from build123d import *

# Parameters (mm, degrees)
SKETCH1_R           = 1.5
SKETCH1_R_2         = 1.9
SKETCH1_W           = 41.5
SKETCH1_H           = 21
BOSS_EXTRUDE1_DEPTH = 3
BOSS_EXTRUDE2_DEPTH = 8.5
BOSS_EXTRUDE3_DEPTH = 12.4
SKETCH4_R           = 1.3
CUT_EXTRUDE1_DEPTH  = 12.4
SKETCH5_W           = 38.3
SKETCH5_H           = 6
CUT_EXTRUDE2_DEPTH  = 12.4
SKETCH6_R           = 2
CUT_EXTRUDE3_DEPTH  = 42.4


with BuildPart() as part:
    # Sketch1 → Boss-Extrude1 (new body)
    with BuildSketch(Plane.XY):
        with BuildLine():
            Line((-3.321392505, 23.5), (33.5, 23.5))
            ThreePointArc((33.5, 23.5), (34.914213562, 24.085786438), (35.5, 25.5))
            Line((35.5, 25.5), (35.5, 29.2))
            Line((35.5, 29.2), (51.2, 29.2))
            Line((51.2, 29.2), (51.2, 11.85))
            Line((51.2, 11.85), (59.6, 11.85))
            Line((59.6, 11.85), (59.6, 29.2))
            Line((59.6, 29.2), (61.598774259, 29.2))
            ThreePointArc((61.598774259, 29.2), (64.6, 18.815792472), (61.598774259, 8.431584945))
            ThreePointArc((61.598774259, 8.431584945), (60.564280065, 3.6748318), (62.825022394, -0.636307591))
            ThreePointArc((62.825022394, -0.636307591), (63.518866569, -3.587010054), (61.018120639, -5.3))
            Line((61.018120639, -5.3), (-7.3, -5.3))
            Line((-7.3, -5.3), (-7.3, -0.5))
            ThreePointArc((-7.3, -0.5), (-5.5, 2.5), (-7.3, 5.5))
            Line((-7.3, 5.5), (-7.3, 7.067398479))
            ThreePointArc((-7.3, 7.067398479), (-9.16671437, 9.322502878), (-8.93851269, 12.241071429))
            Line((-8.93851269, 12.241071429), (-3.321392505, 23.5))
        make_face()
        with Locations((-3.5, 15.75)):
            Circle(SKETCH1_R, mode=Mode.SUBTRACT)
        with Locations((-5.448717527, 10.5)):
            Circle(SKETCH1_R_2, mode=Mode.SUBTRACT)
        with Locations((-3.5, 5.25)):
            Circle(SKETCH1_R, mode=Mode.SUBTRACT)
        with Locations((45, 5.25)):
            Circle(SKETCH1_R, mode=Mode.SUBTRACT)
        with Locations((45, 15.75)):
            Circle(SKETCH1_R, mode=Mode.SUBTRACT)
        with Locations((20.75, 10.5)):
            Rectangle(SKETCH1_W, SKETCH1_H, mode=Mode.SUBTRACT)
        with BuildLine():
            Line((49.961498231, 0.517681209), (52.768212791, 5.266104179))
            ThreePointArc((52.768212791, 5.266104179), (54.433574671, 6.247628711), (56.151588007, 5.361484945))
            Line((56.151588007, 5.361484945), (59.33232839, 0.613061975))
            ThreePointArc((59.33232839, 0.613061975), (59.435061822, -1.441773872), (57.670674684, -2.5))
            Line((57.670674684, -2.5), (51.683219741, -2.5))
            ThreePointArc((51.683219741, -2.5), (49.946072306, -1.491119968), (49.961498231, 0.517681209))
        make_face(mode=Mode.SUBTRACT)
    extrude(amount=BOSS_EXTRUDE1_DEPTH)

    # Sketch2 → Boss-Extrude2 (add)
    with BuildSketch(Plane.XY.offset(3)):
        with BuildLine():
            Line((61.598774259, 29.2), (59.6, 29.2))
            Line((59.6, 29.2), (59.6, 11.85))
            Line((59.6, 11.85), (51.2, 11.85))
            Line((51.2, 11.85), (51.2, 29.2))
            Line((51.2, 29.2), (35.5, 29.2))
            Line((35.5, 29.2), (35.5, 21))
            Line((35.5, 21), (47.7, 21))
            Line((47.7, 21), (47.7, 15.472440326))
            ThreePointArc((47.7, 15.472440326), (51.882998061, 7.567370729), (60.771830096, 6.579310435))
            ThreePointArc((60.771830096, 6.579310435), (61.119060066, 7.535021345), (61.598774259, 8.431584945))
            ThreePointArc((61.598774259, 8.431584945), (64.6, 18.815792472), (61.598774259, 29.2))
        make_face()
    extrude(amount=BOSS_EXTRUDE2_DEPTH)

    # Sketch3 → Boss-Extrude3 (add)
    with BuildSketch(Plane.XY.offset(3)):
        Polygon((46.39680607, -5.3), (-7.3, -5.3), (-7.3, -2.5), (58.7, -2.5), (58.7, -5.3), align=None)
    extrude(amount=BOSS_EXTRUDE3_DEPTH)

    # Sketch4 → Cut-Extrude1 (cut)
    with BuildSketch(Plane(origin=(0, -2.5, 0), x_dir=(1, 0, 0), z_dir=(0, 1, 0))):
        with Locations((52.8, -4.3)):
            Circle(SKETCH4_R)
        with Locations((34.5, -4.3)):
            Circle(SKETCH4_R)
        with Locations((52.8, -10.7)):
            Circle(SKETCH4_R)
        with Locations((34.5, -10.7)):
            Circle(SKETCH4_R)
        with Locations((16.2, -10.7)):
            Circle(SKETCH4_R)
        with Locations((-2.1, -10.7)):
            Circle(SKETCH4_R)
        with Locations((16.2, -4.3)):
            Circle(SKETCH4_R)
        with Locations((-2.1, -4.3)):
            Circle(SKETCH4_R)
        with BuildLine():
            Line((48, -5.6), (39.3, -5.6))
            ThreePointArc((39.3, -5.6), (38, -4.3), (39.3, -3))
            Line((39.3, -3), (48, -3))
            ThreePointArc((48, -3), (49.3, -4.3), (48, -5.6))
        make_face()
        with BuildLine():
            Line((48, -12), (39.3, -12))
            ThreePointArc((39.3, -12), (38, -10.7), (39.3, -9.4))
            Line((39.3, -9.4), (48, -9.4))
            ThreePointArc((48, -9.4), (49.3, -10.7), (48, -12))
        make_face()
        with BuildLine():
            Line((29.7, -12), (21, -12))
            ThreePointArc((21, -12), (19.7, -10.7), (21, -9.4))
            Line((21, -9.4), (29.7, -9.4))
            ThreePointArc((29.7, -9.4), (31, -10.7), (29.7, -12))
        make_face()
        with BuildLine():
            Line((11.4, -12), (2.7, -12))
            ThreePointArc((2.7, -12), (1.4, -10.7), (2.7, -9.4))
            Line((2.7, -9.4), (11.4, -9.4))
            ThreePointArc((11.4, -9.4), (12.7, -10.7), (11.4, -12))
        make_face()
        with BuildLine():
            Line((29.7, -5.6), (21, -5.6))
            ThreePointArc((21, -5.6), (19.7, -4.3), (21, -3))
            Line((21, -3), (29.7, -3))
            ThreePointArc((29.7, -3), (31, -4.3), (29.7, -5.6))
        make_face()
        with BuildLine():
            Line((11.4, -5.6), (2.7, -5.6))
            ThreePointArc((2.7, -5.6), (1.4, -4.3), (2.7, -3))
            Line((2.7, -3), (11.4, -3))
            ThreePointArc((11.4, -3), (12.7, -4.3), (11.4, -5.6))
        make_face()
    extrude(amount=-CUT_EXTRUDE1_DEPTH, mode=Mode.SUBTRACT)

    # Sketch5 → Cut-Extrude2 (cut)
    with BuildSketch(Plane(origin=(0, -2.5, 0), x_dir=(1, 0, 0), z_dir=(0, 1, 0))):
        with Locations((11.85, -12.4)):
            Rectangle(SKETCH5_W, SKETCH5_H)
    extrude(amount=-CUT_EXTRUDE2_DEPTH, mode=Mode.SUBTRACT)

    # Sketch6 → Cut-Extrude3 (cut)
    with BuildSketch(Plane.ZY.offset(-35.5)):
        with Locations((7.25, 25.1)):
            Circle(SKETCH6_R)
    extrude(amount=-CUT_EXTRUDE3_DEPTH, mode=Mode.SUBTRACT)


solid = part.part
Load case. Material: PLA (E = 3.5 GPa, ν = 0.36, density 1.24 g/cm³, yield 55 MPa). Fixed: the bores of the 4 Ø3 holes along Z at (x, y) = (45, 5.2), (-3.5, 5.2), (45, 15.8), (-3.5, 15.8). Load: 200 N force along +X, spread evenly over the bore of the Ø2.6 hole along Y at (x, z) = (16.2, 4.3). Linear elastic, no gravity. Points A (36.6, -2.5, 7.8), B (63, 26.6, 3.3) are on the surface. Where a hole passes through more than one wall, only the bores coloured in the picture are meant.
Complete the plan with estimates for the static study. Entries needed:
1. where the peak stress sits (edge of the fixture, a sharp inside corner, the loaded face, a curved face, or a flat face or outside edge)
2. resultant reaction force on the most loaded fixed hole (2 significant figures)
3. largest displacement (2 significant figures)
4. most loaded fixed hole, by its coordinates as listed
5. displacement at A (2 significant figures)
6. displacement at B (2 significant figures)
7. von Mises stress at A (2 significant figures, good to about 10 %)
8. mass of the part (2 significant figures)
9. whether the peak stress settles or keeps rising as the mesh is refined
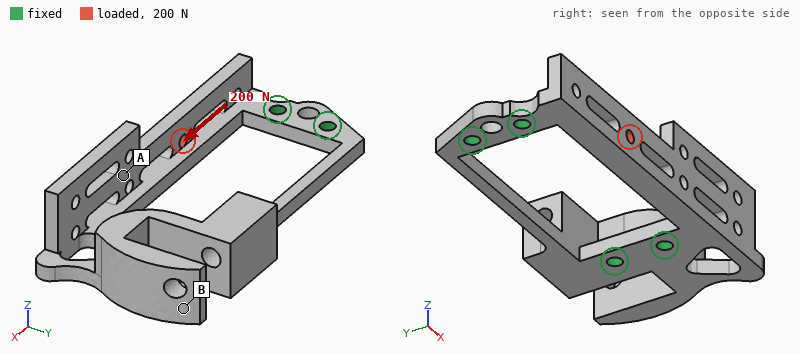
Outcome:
edge of the fixture
160 N
0.13 mm
(45, 5.2)
0.087 mm
0.056 mm
4.2 MPa
8.3 g
keeps rising
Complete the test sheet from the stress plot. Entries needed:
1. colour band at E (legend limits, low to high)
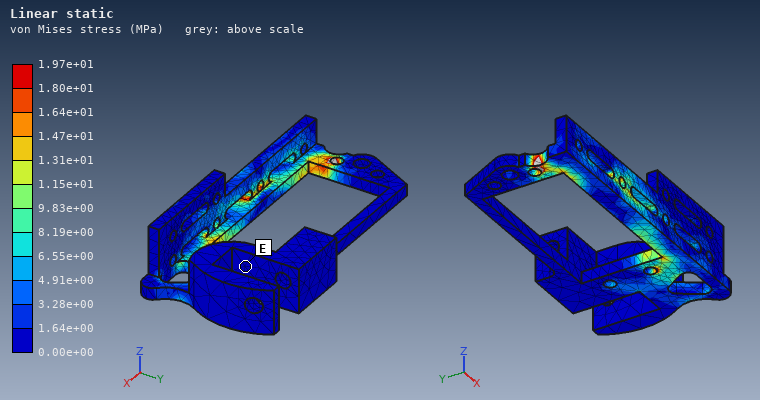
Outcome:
0.00e+00 to 1.64e+00 MPa
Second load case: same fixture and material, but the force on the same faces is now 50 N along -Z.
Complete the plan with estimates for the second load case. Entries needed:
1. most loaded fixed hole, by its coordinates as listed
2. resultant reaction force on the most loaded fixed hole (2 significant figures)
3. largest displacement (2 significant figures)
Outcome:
(-3.5, 5.2)
32 N
0.35 mm
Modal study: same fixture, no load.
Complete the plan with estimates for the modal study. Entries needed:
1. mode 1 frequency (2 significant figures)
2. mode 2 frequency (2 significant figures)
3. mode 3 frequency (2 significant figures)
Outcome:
1300 Hz
1400 Hz
1900 Hz
